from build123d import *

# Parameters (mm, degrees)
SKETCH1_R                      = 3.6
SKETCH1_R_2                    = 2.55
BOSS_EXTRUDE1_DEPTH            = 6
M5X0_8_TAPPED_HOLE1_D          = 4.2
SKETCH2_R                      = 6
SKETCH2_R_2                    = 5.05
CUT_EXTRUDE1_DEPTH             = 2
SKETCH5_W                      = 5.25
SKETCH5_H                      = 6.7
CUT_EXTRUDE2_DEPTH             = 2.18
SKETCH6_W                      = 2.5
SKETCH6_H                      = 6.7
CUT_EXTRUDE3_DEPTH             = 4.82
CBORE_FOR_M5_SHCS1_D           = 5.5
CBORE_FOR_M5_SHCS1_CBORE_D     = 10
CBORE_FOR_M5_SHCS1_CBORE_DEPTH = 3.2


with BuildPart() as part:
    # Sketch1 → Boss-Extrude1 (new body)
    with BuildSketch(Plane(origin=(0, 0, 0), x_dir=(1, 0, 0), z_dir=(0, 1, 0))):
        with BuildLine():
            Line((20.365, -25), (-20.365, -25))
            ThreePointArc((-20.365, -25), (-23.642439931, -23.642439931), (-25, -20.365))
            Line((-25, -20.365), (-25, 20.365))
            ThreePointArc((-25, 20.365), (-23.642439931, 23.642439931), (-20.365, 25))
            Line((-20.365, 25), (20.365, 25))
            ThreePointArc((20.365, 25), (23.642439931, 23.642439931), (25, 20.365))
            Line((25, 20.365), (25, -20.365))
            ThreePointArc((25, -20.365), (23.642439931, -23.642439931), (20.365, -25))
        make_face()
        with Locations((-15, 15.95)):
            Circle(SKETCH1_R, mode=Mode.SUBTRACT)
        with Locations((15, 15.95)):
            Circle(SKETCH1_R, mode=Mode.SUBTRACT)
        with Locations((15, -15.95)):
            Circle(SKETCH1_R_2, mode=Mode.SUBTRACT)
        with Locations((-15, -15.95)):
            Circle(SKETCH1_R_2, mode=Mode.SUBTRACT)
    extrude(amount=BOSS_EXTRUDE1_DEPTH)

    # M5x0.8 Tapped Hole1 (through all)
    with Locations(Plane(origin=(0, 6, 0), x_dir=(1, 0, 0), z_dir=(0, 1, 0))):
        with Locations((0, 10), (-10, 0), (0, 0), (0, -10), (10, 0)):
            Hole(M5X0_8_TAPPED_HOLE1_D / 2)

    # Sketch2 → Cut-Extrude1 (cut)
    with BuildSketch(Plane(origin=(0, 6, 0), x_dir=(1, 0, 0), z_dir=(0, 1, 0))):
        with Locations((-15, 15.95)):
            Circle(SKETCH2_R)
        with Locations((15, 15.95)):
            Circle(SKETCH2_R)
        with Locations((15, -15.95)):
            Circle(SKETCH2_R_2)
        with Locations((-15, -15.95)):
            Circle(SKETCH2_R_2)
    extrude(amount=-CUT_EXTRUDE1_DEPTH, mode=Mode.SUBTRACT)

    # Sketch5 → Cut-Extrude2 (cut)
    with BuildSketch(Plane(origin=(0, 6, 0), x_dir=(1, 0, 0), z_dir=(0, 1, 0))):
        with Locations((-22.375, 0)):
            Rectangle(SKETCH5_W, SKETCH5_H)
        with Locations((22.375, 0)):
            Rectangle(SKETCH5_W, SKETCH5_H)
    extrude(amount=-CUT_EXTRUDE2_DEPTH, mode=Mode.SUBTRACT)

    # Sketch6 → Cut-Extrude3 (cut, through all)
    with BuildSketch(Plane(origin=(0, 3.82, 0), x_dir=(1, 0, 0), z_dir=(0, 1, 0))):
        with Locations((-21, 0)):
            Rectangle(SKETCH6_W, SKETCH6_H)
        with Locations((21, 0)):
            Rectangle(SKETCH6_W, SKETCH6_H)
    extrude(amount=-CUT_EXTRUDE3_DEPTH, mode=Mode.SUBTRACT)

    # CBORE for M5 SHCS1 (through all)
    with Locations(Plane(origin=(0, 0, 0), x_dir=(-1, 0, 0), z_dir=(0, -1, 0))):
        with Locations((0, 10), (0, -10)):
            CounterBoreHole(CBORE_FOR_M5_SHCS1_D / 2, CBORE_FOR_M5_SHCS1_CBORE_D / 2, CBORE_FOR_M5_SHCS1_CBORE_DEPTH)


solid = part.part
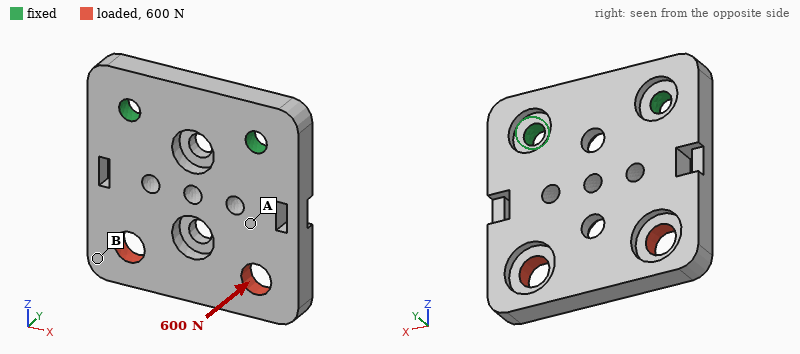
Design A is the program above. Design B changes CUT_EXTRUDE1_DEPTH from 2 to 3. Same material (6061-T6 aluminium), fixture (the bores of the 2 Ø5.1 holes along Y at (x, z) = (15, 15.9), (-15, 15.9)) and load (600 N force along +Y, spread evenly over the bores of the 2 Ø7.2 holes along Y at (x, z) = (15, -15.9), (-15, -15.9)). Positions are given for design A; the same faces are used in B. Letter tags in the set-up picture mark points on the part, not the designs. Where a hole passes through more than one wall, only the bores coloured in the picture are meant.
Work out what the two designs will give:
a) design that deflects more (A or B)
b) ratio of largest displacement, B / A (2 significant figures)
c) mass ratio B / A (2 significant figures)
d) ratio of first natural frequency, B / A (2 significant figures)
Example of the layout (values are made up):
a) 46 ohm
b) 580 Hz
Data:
a) B
b) 1.3
c) 0.98
d) 0.89
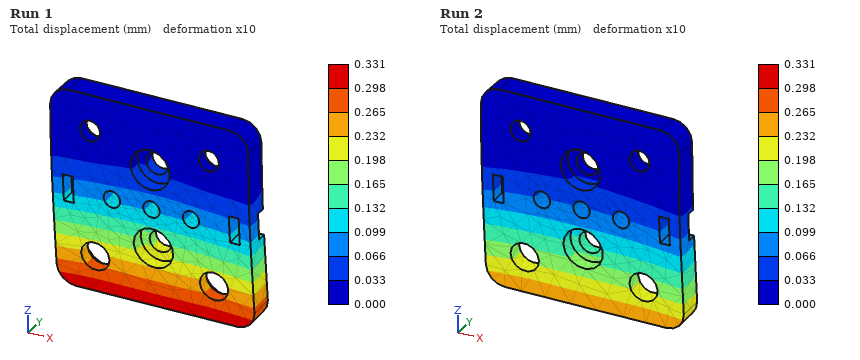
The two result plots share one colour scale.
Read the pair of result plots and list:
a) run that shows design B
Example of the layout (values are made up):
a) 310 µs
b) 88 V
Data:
a) Run 1
